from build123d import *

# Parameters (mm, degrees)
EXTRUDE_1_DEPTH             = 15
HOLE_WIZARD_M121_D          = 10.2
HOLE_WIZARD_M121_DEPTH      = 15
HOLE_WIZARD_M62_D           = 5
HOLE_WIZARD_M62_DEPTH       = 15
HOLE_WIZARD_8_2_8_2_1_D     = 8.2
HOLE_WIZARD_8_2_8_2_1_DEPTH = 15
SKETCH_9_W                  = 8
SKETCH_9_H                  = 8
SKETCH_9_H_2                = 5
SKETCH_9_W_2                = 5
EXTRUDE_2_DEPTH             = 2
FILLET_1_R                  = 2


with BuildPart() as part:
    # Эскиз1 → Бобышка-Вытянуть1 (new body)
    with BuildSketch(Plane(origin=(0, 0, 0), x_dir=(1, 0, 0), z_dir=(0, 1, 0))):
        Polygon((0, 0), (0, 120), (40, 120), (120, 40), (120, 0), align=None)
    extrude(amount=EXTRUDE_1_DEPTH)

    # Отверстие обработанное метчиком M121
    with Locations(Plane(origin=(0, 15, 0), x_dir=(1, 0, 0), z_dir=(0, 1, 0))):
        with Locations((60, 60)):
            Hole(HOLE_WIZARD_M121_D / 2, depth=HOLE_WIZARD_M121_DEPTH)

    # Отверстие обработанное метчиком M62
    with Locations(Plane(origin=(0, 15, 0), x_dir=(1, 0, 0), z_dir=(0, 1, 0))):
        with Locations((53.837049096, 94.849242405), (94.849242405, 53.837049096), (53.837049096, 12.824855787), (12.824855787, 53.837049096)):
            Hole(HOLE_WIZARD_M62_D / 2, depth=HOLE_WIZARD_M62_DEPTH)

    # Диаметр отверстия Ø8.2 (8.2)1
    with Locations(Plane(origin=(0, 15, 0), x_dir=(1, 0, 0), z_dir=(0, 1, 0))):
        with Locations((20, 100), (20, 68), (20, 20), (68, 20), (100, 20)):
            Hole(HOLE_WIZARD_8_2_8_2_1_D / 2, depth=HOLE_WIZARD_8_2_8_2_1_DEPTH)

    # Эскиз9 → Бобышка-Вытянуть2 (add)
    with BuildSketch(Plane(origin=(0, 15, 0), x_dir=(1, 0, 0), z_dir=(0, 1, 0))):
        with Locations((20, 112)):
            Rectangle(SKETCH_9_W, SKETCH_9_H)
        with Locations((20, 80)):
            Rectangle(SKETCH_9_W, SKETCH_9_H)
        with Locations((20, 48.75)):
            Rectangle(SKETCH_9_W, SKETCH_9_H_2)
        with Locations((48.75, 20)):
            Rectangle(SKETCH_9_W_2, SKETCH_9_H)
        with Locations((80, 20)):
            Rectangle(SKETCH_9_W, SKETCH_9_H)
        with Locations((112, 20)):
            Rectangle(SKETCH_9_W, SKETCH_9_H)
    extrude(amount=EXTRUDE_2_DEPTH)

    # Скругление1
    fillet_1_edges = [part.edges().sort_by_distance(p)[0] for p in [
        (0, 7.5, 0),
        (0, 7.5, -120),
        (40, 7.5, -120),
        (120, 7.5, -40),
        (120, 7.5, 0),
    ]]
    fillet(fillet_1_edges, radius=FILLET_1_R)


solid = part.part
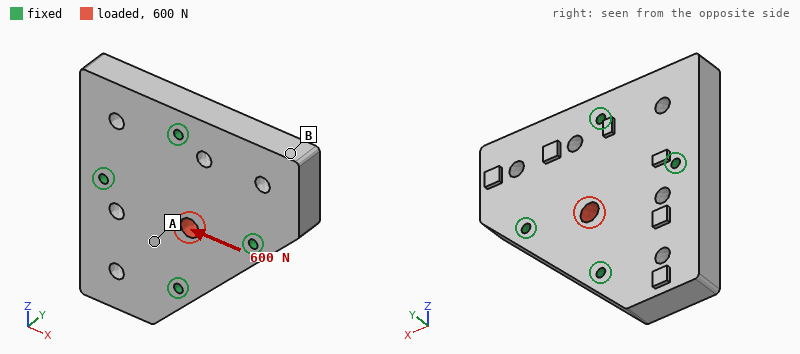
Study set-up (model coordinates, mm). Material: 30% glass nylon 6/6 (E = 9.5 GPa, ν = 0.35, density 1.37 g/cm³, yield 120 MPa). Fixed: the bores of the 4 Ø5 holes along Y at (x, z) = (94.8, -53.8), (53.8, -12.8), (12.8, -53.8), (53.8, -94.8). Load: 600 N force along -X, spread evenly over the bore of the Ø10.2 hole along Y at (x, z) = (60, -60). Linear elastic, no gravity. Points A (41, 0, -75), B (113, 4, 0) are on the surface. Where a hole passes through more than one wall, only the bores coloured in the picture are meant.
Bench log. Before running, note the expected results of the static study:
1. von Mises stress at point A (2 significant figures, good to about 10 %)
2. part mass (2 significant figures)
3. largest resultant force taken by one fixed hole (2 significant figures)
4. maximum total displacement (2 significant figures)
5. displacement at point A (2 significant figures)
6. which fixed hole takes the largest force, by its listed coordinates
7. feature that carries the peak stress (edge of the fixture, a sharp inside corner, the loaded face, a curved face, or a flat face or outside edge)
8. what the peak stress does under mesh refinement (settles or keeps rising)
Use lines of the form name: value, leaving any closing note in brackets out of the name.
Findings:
von Mises stress at point A: 0.36 MPa
part mass: 220 g
largest resultant force taken by one fixed hole: 230 N
maximum total displacement: 3.4 µm
displacement at point A: 1.5 µm
which fixed hole takes the largest force, by its listed coordinates: (94.8, -53.8)
feature that carries the peak stress: edge of the fixture
what the peak stress does under mesh refinement: keeps rising
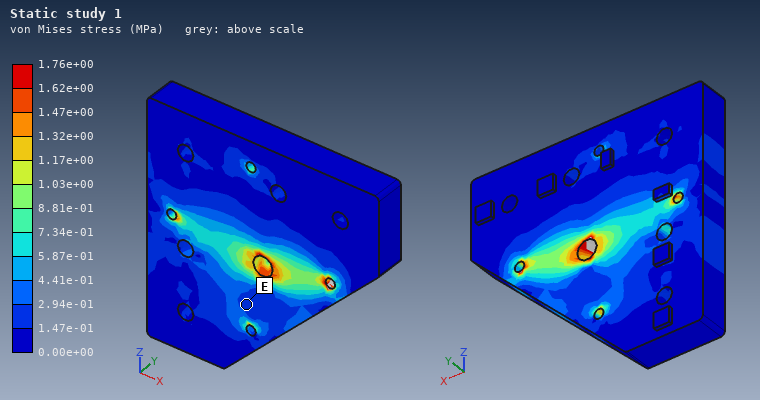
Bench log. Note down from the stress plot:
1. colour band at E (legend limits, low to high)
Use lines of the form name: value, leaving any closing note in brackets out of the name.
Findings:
colour band at E: 1.47e-01 to 2.94e-01 MPa
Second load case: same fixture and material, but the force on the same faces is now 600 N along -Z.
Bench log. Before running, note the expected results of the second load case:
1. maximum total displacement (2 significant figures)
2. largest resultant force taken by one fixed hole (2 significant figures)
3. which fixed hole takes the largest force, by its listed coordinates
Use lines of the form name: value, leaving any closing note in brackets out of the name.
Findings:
maximum total displacement: 3.4 µm
largest resultant force taken by one fixed hole: 230 N
which fixed hole takes the largest force, by its listed coordinates: (53.8, -94.8)
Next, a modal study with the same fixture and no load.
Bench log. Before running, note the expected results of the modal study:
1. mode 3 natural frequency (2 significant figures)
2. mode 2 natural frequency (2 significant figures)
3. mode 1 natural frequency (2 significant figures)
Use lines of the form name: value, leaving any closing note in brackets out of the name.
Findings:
mode 3 natural frequency: 3600 Hz
mode 2 natural frequency: 2600 Hz
mode 1 natural frequency: 2600 Hz
